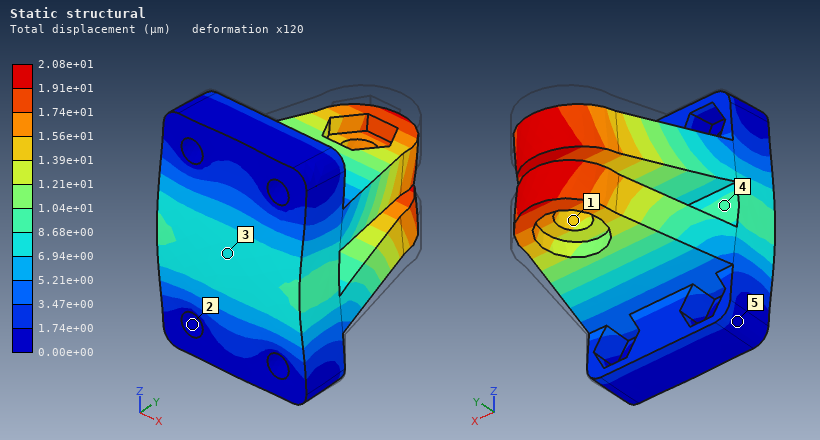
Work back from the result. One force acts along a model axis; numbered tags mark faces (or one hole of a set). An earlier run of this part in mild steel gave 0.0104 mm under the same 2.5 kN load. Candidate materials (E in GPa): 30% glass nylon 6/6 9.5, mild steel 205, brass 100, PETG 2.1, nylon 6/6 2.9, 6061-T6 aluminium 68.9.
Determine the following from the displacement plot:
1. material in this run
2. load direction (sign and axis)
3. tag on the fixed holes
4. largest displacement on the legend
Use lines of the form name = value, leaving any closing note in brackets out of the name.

material in this run = brass
load direction = -Y
tag on the fixed holes = 2
largest displacement on the legend = 2.08e+01 µm
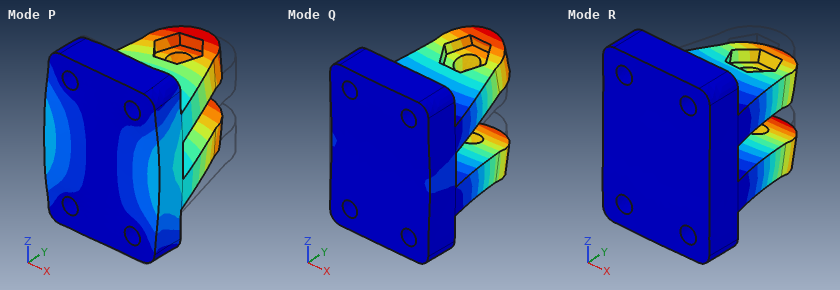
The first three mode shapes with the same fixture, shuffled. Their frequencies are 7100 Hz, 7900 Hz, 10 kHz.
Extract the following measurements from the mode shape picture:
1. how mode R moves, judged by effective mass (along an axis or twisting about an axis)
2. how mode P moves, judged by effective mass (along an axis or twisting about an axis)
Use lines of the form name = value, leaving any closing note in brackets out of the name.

how mode R moves, judged by effective mass = along Z
how mode P moves, judged by effective mass = along X
